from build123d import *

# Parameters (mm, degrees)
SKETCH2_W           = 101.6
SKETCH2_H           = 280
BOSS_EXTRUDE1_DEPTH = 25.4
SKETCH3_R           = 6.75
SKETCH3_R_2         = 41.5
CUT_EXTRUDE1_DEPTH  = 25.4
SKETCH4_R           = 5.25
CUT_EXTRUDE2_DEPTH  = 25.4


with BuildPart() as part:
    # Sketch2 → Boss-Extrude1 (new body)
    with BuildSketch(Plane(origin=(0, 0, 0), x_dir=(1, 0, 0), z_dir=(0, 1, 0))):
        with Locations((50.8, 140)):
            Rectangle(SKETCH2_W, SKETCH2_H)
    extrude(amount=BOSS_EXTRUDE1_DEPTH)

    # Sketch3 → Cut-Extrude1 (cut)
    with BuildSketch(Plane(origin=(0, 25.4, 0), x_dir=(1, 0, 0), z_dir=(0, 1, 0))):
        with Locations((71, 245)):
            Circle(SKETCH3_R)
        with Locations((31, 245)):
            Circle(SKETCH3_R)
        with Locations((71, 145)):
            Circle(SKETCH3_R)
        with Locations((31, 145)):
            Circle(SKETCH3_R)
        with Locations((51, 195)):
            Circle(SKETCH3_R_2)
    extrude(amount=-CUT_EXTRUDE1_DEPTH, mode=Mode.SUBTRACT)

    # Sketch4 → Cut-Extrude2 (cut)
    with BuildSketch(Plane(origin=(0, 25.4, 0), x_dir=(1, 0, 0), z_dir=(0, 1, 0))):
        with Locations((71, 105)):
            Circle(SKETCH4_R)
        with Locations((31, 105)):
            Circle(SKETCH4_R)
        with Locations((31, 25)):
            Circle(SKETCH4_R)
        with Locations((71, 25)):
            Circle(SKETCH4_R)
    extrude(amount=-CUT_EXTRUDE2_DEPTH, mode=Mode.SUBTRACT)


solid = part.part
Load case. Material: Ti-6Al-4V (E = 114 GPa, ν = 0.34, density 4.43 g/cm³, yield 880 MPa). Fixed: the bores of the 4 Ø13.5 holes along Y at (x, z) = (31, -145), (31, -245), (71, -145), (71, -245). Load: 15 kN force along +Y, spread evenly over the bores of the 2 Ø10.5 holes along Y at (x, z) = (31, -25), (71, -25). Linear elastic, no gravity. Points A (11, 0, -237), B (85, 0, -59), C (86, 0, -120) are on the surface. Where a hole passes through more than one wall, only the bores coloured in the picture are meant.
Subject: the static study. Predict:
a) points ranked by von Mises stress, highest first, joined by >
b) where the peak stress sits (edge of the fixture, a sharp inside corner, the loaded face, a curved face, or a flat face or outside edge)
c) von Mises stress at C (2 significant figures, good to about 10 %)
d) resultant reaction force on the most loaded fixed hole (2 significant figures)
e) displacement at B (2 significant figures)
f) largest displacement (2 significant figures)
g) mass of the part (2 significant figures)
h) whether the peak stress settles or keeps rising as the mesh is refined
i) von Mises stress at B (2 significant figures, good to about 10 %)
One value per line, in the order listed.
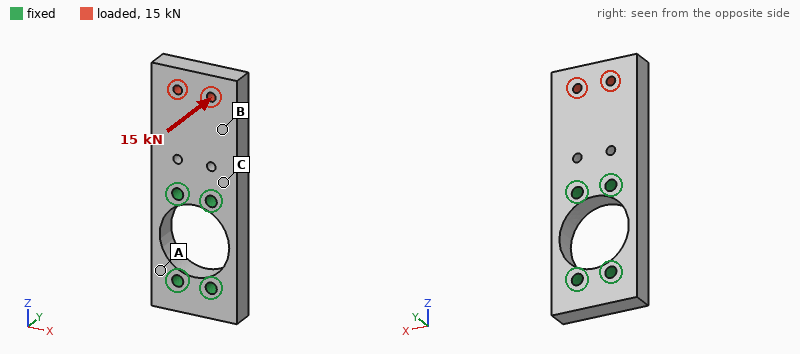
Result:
C > B > A
edge of the fixture
130 MPa
8.4 kN
0.35 mm
0.77 mm
2.5 kg
keeps rising
48 MPa
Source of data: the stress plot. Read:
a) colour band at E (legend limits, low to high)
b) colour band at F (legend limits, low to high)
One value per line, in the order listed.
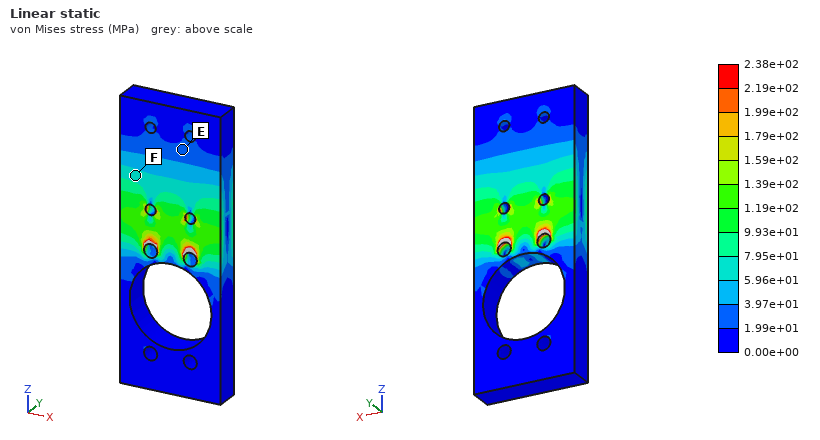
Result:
1.99e+01 to 3.97e+01 MPa
5.96e+01 to 7.95e+01 MPa
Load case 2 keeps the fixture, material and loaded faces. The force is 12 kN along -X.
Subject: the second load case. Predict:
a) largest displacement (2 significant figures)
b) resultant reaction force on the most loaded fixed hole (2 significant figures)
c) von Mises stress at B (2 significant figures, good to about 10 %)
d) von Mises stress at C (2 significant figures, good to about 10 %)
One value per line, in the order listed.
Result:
79 µm
23 kN
9.6 MPa
20 MPa
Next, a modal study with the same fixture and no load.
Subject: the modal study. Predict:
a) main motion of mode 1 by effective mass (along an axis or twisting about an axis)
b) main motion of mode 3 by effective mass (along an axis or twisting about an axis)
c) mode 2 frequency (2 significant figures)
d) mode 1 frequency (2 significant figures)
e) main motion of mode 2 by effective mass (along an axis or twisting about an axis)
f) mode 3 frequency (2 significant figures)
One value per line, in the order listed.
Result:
along Y
twisting about Z
2500 Hz
970 Hz
along X
2600 Hz
